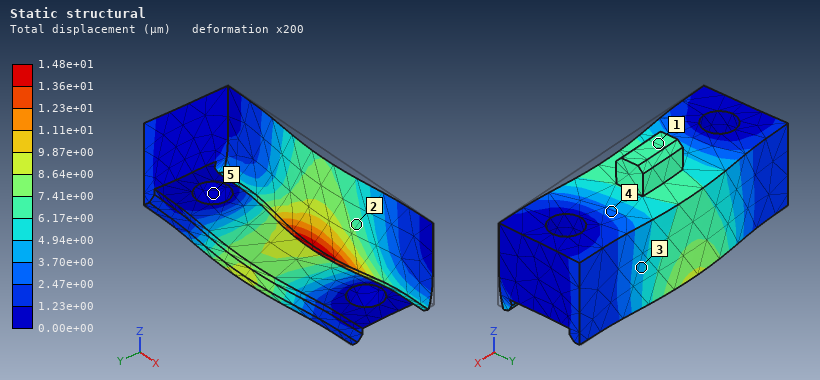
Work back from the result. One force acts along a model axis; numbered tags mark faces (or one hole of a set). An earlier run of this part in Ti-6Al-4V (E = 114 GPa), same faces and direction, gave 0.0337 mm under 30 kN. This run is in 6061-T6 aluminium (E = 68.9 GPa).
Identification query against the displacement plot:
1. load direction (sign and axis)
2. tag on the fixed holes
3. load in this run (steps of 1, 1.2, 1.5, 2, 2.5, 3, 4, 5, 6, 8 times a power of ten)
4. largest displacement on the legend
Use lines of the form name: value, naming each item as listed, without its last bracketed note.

load direction: +Y
tag on the fixed holes: 5
load in this run: 8 kN
largest displacement on the legend: 1.48e+01 µm
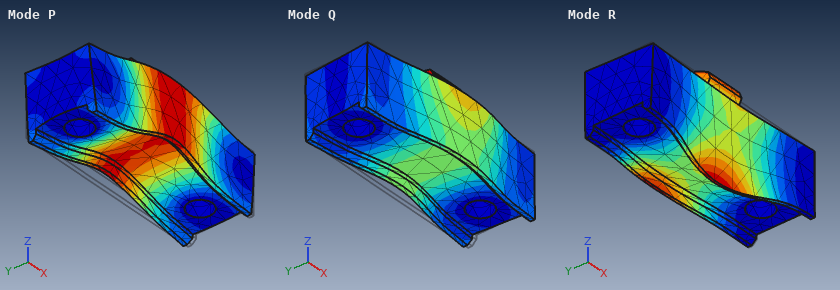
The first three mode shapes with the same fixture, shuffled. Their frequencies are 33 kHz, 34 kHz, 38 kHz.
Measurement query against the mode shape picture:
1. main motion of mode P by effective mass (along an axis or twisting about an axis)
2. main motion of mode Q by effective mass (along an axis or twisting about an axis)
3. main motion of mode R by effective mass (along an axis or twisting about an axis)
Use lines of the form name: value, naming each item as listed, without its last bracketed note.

main motion of mode P by effective mass: along Z
main motion of mode Q by effective mass: along Y
main motion of mode R by effective mass: twisting about X
